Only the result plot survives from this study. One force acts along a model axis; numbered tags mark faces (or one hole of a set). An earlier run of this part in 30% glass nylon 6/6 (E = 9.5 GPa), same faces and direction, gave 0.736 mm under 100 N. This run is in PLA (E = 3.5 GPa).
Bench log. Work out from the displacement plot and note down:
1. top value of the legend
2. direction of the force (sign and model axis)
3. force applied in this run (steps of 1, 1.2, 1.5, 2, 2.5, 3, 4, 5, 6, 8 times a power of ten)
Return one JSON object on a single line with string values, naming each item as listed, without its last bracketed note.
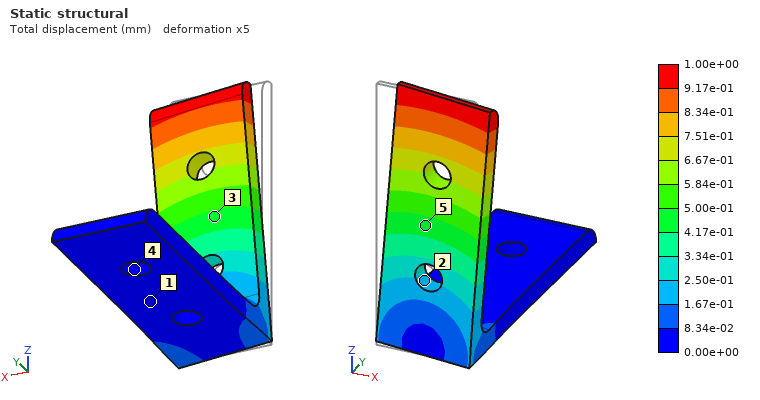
{"top value of the legend": "1.00e+00 mm", "direction of the force": "+X", "force applied in this run": "50 N"}
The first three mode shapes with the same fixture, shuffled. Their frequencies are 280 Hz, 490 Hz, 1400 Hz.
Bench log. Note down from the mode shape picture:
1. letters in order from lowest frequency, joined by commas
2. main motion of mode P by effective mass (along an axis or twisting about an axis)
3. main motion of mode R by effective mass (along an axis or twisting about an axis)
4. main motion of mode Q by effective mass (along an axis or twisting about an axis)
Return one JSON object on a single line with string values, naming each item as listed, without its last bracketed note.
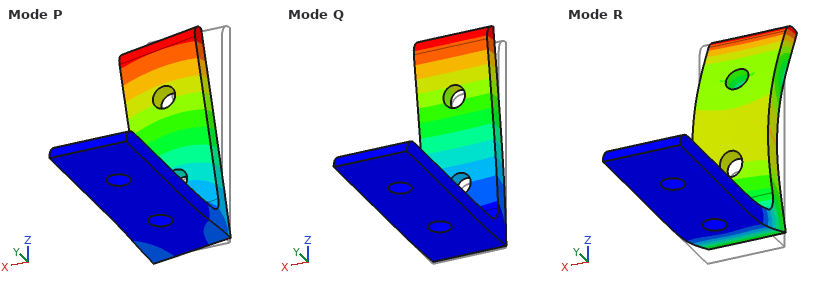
{"letters in order from lowest frequency, joined by commas": "Q, P, R", "main motion of mode P by effective mass": "along X", "main motion of mode R by effective mass": "along Z", "main motion of mode Q by effective mass": "along Y"}
